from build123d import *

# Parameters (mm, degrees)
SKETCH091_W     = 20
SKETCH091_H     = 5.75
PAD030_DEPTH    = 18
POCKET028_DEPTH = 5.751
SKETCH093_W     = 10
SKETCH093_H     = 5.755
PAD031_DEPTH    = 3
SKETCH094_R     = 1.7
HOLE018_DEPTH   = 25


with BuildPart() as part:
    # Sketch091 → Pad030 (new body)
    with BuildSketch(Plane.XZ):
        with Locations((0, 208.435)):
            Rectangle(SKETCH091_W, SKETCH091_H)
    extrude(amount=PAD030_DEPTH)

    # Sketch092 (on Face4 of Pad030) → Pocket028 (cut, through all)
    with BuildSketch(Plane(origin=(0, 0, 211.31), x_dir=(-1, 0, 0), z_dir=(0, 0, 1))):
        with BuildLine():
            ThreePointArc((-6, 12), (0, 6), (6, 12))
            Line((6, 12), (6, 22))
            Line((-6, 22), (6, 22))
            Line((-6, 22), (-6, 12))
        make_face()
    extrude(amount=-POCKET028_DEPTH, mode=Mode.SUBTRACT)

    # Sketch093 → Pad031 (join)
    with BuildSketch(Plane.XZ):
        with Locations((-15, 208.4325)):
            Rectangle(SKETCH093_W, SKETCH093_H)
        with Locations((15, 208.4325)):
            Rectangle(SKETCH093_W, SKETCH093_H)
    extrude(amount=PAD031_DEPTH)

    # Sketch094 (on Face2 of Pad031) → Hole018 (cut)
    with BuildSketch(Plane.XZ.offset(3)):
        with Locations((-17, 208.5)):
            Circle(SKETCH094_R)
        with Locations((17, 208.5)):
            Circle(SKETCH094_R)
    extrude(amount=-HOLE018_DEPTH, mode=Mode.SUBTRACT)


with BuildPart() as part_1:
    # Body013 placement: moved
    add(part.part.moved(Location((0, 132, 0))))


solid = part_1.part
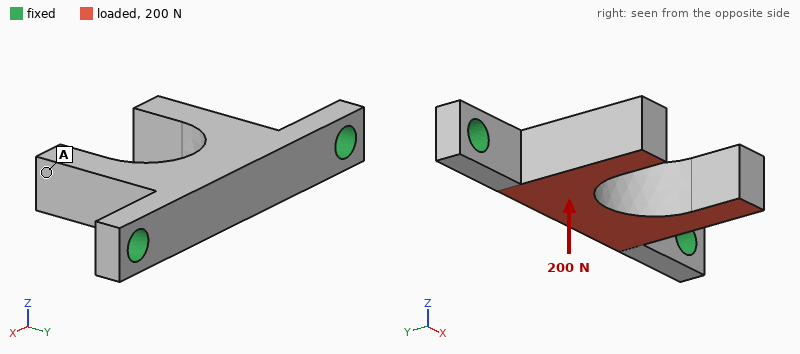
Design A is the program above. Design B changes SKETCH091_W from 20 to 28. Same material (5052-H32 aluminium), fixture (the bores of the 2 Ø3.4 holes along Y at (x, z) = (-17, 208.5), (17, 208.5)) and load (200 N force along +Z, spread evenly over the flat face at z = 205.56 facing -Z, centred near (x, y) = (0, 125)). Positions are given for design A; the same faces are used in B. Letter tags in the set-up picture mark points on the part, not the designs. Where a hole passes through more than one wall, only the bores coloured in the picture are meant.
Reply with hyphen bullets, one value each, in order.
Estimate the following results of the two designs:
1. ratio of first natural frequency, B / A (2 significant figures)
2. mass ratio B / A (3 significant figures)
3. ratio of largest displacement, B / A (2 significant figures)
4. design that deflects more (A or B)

- 1.1
- 1.43
- 0.50
- A
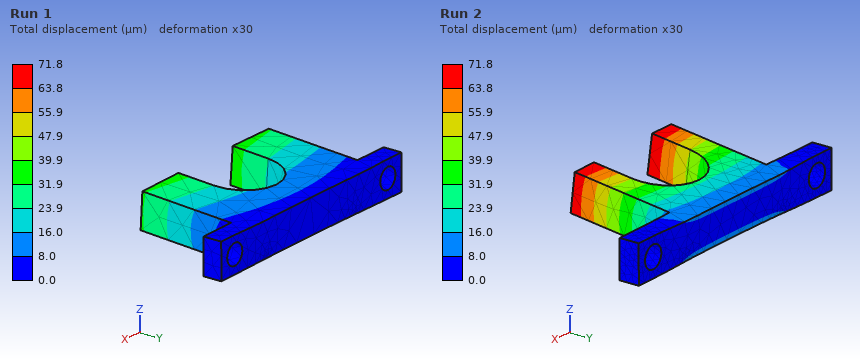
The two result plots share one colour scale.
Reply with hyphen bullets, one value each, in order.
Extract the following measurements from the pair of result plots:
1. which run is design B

- Run 1
